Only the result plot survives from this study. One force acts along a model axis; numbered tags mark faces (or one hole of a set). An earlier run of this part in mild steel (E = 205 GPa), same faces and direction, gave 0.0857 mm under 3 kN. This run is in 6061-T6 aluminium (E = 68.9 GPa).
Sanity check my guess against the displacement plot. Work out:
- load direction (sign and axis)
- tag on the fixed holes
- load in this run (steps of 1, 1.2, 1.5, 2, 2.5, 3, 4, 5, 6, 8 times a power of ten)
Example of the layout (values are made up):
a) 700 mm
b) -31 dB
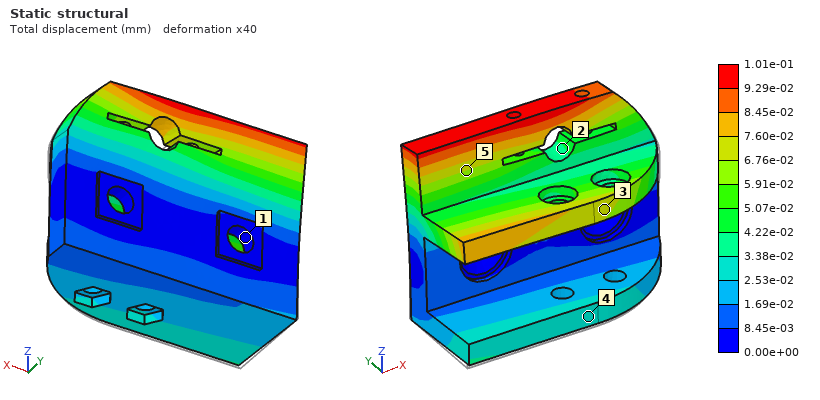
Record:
a) +Y
b) 1
c) 1.2 kN
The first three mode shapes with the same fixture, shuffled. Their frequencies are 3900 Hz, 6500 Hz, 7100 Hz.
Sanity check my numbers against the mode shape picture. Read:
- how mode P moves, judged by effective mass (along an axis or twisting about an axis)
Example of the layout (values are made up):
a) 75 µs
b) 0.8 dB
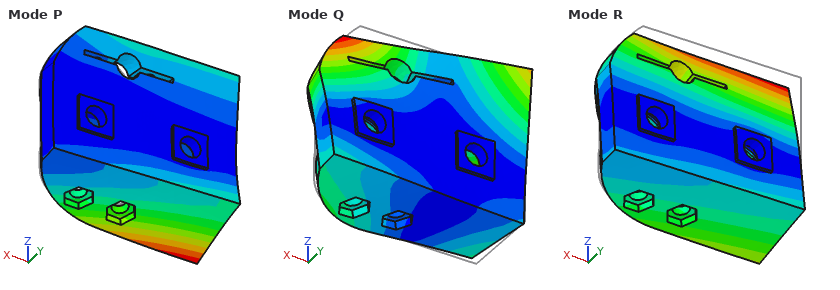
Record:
a) along Y
